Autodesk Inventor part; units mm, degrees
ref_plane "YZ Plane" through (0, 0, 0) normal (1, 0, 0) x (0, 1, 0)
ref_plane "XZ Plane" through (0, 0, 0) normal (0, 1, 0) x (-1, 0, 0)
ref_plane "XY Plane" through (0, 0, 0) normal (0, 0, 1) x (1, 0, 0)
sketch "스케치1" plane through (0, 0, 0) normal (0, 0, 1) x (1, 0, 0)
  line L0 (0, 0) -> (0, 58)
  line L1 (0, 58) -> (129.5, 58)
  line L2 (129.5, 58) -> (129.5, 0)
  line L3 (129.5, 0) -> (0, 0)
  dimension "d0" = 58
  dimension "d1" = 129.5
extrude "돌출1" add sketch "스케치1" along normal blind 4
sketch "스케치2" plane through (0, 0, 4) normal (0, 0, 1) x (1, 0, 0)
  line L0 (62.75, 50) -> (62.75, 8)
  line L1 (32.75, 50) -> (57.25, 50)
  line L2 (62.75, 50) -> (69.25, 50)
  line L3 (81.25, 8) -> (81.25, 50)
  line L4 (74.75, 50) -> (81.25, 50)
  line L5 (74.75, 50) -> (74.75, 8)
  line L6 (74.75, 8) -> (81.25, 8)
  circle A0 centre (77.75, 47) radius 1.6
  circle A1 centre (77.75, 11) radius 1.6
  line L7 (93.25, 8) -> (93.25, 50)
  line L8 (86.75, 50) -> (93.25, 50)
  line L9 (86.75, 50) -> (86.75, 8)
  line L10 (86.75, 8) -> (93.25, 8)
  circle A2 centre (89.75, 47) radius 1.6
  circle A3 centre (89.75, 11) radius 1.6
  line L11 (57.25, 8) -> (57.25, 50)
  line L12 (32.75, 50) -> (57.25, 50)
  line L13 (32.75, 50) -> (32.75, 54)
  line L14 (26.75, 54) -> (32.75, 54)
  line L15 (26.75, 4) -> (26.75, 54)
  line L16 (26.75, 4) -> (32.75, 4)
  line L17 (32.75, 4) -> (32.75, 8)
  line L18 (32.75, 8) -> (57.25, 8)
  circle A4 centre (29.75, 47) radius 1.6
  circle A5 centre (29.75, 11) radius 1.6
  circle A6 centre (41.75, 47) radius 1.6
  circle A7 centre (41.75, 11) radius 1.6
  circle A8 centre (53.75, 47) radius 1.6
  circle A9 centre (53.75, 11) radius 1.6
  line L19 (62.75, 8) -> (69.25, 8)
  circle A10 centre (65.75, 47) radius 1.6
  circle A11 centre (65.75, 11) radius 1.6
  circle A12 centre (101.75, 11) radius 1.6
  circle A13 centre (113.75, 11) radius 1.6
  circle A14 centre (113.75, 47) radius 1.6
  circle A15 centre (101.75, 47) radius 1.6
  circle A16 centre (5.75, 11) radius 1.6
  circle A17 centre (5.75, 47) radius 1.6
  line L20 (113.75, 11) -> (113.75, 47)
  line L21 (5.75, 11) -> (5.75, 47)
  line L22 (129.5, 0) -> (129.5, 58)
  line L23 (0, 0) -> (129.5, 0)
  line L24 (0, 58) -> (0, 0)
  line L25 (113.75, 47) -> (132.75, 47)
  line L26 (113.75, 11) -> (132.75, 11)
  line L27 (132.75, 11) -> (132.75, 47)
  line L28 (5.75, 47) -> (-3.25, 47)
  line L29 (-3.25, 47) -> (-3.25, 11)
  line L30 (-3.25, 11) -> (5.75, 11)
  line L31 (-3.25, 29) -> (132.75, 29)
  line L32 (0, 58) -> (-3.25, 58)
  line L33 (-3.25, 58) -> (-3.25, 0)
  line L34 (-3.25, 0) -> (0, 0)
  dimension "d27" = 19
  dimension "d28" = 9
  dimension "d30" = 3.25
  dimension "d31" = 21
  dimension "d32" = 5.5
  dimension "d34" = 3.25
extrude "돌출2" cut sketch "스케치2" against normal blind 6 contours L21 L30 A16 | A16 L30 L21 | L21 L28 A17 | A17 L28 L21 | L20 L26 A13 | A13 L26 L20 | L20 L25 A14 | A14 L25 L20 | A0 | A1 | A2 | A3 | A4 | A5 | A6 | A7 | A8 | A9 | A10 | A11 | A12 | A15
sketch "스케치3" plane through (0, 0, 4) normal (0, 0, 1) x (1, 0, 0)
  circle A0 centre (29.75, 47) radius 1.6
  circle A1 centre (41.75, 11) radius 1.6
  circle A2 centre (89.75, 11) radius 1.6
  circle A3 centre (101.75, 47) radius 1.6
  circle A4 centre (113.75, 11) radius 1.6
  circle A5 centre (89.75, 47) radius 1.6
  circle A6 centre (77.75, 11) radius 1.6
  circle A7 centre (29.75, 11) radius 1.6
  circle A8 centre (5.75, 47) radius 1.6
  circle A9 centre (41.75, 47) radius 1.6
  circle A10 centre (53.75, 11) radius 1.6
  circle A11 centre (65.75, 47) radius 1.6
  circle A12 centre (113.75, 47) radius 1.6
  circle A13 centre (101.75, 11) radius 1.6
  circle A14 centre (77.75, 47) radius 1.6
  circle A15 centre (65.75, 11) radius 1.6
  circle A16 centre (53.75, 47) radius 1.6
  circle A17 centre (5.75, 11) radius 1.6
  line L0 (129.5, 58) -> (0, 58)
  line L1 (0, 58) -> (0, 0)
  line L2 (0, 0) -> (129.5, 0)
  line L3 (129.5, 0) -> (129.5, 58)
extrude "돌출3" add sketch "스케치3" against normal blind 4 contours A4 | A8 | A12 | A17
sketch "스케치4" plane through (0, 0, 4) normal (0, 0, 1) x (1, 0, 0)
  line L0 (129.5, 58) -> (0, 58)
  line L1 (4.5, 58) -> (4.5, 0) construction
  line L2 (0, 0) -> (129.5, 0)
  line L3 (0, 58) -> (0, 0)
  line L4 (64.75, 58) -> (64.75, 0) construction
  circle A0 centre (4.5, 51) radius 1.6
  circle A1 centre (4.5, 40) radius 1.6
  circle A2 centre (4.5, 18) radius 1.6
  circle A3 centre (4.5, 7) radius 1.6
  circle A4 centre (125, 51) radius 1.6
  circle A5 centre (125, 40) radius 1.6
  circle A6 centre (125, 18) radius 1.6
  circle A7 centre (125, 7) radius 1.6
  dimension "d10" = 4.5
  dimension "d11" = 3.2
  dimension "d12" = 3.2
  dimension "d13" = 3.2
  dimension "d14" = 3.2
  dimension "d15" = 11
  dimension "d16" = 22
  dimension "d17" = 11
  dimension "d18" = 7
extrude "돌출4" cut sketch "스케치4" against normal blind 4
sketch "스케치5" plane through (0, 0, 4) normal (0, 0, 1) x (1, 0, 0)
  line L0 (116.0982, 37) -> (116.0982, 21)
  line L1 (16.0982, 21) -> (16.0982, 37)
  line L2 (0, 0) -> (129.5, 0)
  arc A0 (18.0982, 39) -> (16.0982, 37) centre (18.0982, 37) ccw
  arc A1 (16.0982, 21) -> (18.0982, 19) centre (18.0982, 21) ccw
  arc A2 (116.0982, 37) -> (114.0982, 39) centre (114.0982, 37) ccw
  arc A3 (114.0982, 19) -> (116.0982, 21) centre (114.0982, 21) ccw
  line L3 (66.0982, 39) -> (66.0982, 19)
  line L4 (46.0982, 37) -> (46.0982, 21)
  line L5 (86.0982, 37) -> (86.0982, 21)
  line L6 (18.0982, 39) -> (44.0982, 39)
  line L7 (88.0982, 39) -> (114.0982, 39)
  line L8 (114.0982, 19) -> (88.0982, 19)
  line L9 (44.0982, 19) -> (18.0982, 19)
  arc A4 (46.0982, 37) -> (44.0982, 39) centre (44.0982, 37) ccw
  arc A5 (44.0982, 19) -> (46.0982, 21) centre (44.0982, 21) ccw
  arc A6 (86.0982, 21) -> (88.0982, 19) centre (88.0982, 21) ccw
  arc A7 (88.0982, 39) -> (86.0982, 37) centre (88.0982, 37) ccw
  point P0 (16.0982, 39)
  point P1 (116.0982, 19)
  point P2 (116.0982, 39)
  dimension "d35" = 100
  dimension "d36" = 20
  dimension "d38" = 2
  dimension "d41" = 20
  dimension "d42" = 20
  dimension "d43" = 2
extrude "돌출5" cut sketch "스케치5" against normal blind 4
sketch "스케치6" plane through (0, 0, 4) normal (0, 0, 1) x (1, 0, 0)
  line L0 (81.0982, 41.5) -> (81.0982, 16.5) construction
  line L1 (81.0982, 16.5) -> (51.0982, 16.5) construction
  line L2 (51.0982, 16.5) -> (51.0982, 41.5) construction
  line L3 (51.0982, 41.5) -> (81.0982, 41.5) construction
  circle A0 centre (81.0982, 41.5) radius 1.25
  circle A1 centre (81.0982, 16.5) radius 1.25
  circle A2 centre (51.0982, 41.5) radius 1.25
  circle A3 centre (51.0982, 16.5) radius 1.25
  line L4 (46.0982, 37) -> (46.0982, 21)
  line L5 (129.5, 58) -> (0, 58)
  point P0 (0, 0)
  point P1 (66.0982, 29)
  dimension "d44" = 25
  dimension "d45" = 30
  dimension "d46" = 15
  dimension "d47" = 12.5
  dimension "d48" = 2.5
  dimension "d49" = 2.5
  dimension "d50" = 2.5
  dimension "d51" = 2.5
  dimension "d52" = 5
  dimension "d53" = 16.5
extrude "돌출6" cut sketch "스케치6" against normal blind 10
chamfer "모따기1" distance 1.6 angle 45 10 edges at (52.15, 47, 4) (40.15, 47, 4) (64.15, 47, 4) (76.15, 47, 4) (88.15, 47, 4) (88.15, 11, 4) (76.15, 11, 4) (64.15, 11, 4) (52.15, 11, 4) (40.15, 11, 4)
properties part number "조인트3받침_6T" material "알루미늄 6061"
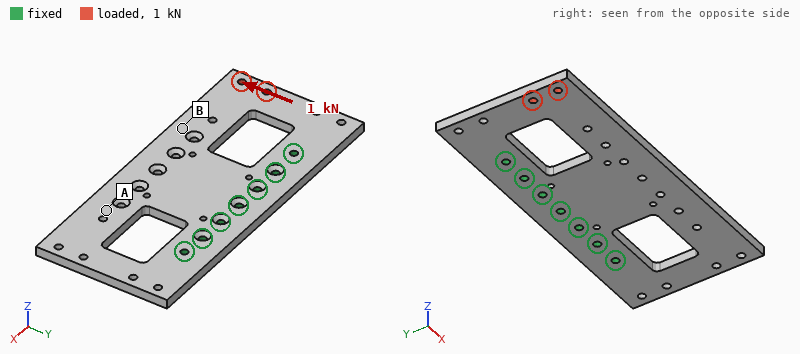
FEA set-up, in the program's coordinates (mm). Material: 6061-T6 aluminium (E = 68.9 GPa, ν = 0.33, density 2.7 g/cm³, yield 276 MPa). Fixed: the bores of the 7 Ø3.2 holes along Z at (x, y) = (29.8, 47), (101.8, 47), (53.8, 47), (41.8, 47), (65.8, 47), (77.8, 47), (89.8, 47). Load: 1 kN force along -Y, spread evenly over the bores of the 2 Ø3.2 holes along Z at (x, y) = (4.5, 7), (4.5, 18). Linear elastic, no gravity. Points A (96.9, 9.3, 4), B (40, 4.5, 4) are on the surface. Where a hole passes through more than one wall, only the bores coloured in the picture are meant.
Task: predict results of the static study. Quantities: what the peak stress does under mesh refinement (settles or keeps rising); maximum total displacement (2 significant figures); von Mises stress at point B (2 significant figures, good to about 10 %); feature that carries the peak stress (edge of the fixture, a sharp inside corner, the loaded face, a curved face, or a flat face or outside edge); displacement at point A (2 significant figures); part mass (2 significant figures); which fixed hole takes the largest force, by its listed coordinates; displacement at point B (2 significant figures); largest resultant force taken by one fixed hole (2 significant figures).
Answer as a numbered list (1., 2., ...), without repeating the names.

1. keeps rising
2. 41 µm
3. 9.6 MPa
4. edge of the fixture
5. 8.7 µm
6. 66 g
7. (29.8, 47)
8. 17 µm
9. 1.3 kN
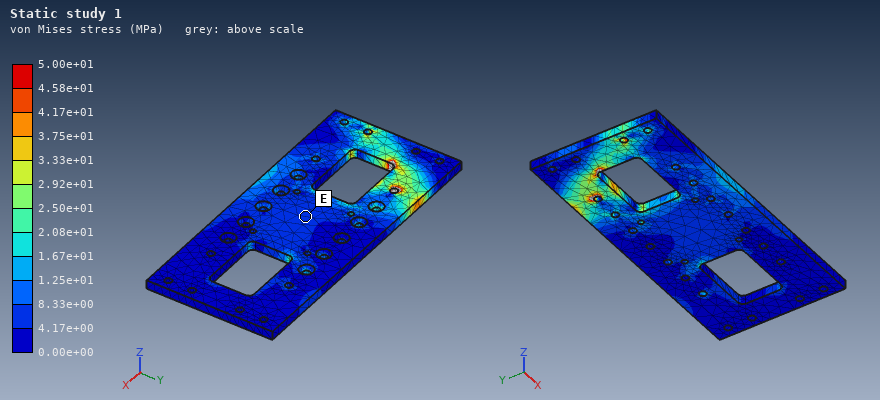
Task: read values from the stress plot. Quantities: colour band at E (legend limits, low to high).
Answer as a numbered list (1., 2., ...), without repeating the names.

1. 4.17e+00 to 8.33e+00 MPa
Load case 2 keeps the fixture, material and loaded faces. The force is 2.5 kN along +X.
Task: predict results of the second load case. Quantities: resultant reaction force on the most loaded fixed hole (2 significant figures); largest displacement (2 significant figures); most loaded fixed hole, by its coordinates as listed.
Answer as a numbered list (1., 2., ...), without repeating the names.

1. 900 N
2. 66 µm
3. (29.8, 47)
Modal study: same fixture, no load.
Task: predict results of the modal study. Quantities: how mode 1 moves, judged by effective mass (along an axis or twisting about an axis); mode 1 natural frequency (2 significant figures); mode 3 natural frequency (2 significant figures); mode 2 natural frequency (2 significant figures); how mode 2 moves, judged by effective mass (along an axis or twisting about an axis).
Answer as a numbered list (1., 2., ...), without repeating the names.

1. along Z
2. 980 Hz
3. 2000 Hz
4. 1200 Hz
5. twisting about Y
